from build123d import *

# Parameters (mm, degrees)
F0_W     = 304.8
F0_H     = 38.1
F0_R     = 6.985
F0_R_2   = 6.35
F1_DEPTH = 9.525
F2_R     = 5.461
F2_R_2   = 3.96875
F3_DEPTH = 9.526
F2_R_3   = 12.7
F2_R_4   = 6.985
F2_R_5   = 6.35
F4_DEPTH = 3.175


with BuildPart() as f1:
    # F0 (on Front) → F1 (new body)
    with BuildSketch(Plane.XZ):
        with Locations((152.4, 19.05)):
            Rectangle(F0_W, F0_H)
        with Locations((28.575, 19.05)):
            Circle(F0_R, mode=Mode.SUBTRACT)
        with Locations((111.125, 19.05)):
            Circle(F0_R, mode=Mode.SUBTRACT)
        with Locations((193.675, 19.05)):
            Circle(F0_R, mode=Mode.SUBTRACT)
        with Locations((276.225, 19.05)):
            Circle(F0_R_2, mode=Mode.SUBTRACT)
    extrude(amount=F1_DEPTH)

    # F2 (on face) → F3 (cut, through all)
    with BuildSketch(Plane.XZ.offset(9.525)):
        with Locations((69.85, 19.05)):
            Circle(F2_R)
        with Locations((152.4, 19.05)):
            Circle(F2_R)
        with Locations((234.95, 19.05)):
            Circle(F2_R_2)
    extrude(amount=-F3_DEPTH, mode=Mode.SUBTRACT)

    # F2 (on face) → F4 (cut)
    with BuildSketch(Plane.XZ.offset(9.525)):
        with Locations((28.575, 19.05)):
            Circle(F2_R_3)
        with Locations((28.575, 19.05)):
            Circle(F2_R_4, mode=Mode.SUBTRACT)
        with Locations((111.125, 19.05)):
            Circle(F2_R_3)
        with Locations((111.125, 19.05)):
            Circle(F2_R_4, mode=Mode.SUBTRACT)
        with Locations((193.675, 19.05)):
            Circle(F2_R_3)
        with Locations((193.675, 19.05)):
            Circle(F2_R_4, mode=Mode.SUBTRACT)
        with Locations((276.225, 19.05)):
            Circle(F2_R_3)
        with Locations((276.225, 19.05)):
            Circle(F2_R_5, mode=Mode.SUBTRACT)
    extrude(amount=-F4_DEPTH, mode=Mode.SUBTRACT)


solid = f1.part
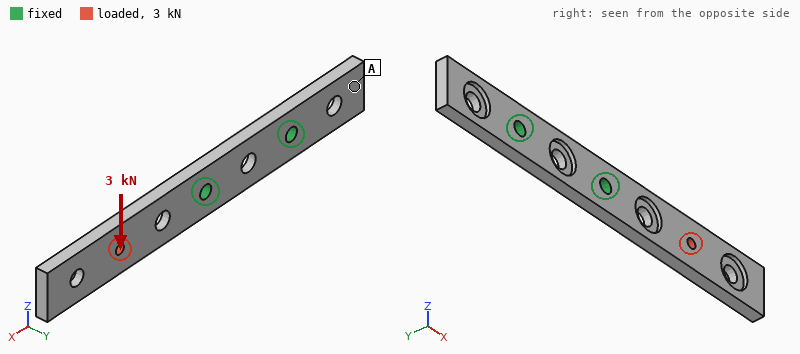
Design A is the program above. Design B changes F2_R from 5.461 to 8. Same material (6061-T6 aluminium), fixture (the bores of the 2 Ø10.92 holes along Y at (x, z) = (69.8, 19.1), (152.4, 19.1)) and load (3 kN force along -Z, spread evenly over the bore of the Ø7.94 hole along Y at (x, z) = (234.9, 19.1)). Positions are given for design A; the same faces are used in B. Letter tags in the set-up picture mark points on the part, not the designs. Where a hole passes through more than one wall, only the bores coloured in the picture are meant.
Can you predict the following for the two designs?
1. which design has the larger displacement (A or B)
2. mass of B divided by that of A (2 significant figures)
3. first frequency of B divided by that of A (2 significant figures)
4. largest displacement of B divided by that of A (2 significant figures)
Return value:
A
0.98
1.0
0.84
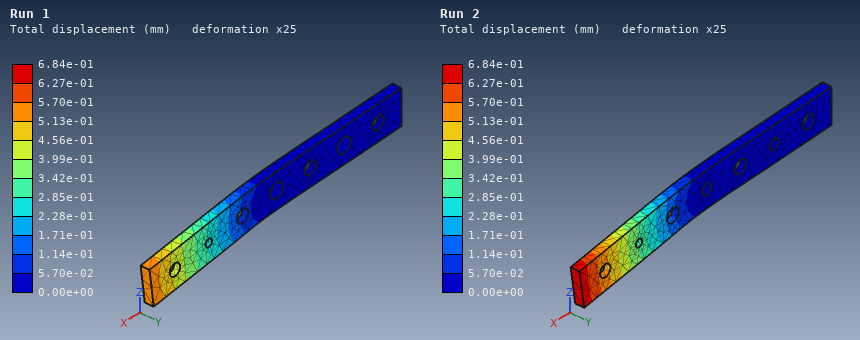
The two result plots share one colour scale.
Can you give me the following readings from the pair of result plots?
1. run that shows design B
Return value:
Run 1
